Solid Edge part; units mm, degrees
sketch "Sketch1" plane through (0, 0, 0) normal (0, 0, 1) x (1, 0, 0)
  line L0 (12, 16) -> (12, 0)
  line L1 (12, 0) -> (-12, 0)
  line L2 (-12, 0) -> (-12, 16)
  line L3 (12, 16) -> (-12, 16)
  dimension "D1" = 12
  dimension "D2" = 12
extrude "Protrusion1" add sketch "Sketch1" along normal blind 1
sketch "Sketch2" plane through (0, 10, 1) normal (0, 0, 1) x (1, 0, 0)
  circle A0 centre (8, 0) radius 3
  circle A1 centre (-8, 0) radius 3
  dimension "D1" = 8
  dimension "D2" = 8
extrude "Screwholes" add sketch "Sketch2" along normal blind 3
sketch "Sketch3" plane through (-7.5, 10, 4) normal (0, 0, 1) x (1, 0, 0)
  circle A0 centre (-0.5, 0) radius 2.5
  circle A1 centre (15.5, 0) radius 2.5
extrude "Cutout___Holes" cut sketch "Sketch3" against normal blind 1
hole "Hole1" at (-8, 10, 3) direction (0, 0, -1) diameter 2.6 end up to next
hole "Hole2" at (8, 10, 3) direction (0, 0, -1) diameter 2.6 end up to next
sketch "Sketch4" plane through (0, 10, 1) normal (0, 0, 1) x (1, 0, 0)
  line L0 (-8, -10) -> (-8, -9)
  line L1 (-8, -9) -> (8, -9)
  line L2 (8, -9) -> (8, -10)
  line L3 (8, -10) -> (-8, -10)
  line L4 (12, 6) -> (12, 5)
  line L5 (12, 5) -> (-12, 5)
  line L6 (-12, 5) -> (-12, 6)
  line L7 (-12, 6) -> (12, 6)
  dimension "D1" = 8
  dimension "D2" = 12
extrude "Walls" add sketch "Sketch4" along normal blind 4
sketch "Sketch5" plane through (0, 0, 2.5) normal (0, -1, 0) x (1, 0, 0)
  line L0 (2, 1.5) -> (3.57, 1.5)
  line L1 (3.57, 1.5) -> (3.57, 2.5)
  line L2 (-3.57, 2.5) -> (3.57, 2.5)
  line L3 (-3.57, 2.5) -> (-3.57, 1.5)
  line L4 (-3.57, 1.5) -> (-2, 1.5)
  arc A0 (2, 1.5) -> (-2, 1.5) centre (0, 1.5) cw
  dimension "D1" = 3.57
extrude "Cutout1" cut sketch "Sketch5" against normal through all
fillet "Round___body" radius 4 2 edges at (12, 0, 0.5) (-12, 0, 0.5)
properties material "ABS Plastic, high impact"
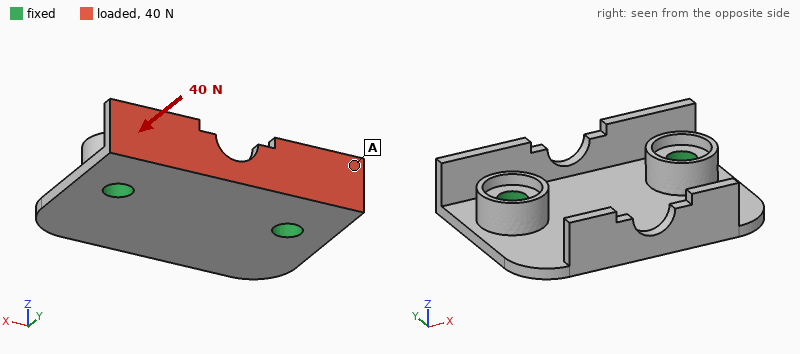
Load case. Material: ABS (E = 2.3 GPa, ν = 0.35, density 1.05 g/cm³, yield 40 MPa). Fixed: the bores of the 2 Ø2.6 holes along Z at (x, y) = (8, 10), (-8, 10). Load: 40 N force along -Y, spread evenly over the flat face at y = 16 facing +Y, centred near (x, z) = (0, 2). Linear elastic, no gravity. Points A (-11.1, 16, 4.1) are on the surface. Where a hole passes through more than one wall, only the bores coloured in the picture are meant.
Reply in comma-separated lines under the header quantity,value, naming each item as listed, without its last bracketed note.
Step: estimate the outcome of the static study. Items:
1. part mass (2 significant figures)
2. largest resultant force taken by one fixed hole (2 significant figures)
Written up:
quantity,value
part mass,0.64 g
largest resultant force taken by one fixed hole,20 N
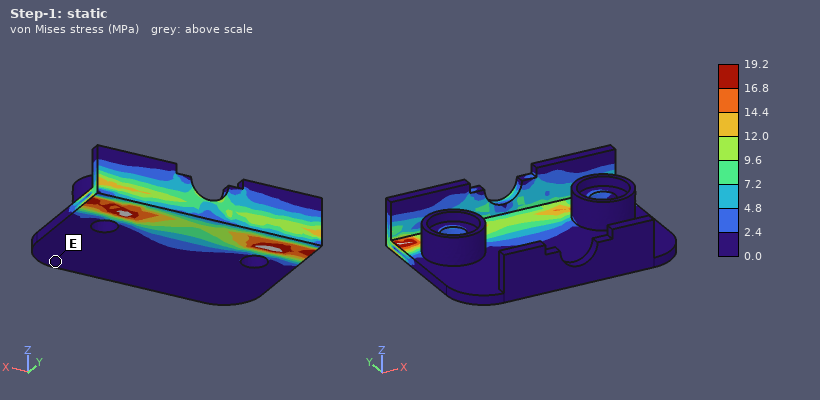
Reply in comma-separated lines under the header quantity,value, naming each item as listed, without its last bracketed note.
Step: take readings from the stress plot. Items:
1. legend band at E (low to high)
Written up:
quantity,value
legend band at E,0.0 to 2.4 MPa
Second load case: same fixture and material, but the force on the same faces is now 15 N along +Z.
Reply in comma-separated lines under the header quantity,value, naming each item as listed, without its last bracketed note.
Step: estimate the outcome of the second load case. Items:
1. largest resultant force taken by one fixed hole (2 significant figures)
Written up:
quantity,value
largest resultant force taken by one fixed hole,7.5 N
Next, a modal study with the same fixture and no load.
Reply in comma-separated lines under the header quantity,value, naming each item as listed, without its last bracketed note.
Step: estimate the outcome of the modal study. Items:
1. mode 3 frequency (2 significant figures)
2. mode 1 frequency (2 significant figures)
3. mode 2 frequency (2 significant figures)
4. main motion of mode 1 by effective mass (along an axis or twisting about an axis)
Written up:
quantity,value
mode 3 frequency,5100 Hz
mode 1 frequency,2400 Hz
mode 2 frequency,4000 Hz
main motion of mode 1 by effective mass,along Z
